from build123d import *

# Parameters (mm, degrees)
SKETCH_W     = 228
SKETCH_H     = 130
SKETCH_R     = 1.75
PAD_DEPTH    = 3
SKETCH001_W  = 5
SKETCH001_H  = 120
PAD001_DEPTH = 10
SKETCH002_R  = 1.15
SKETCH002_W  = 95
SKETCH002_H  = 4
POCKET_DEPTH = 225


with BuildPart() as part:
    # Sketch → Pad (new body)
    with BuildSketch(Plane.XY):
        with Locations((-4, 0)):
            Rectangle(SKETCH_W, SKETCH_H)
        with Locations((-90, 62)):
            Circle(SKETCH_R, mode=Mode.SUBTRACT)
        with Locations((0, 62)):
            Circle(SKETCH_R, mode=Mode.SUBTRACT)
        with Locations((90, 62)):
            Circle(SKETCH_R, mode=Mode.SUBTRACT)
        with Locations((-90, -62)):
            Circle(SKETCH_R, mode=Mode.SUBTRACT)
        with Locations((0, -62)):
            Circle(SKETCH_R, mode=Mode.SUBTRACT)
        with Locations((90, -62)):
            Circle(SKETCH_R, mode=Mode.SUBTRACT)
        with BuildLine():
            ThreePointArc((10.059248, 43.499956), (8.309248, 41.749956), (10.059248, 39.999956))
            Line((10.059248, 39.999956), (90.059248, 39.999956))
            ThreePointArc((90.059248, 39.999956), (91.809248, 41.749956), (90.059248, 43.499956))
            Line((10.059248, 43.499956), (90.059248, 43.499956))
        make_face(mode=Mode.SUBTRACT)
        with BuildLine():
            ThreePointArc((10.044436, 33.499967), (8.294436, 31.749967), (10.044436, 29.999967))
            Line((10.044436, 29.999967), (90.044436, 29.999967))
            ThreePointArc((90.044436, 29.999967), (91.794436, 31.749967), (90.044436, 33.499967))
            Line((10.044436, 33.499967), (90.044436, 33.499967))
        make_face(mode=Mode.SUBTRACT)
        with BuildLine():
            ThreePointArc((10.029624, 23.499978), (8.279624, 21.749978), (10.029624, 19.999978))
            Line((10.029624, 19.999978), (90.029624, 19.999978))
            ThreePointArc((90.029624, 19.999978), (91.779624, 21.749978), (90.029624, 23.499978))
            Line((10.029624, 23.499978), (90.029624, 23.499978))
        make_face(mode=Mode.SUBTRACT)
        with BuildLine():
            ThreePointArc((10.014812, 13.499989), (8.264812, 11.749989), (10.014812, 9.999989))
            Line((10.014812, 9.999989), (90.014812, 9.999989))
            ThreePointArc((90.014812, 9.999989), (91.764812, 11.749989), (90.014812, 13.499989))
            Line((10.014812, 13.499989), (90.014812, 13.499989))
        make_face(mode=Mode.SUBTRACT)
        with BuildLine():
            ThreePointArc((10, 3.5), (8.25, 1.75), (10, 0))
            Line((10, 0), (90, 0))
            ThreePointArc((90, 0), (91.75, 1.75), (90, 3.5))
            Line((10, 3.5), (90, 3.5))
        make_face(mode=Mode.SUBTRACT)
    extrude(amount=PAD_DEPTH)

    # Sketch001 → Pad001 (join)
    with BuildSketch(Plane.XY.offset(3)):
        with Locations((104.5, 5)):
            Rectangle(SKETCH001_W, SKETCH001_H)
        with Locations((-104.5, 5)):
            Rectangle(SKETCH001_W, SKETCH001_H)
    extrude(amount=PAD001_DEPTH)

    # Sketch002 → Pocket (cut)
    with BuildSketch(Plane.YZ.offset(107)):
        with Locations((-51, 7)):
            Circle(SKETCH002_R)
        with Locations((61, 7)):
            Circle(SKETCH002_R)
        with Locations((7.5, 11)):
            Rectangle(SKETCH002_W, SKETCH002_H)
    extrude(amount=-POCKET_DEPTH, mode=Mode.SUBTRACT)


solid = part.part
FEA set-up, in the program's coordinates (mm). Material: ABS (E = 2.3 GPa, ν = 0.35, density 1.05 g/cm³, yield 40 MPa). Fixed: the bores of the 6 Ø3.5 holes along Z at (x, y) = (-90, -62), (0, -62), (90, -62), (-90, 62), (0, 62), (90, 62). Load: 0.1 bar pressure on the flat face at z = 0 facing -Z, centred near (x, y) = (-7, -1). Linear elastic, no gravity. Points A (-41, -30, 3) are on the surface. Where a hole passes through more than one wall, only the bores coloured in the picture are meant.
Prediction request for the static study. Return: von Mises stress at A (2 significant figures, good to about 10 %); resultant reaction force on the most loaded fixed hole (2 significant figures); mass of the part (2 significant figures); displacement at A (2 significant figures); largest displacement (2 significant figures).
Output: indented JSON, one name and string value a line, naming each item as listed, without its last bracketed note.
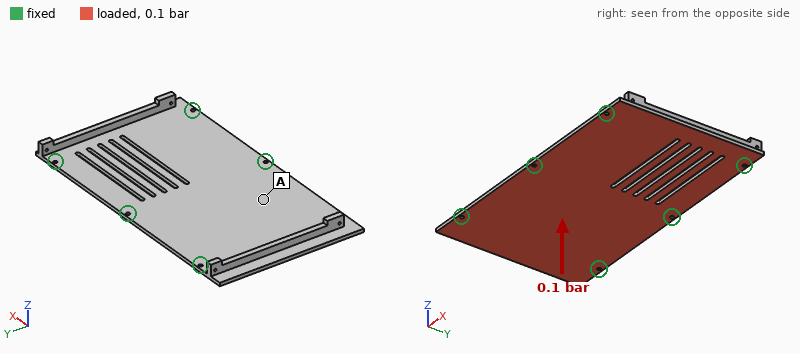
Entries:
{
  "von Mises stress at A": "3.4 MPa",
  "resultant reaction force on the most loaded fixed hole": "63 N",
  "mass of the part": "97 g",
  "displacement at A": "1.5 mm",
  "largest displacement": "3.0 mm"
}
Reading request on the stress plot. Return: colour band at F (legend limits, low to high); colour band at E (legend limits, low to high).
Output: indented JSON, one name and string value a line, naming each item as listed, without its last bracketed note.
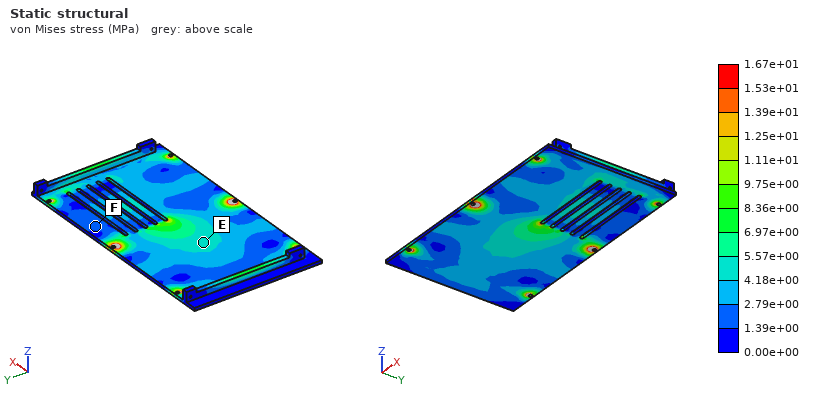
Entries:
{
  "colour band at F": "1.39e+00 to 2.79e+00 MPa",
  "colour band at E": "4.18e+00 to 5.57e+00 MPa"
}
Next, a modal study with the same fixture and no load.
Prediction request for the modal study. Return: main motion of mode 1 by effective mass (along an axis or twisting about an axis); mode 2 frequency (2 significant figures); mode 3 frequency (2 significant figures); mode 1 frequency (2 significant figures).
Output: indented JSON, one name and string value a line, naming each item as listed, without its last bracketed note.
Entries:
{
  "main motion of mode 1 by effective mass": "along Z",
  "mode 2 frequency": "290 Hz",
  "mode 3 frequency": "350 Hz",
  "mode 1 frequency": "220 Hz"
}
